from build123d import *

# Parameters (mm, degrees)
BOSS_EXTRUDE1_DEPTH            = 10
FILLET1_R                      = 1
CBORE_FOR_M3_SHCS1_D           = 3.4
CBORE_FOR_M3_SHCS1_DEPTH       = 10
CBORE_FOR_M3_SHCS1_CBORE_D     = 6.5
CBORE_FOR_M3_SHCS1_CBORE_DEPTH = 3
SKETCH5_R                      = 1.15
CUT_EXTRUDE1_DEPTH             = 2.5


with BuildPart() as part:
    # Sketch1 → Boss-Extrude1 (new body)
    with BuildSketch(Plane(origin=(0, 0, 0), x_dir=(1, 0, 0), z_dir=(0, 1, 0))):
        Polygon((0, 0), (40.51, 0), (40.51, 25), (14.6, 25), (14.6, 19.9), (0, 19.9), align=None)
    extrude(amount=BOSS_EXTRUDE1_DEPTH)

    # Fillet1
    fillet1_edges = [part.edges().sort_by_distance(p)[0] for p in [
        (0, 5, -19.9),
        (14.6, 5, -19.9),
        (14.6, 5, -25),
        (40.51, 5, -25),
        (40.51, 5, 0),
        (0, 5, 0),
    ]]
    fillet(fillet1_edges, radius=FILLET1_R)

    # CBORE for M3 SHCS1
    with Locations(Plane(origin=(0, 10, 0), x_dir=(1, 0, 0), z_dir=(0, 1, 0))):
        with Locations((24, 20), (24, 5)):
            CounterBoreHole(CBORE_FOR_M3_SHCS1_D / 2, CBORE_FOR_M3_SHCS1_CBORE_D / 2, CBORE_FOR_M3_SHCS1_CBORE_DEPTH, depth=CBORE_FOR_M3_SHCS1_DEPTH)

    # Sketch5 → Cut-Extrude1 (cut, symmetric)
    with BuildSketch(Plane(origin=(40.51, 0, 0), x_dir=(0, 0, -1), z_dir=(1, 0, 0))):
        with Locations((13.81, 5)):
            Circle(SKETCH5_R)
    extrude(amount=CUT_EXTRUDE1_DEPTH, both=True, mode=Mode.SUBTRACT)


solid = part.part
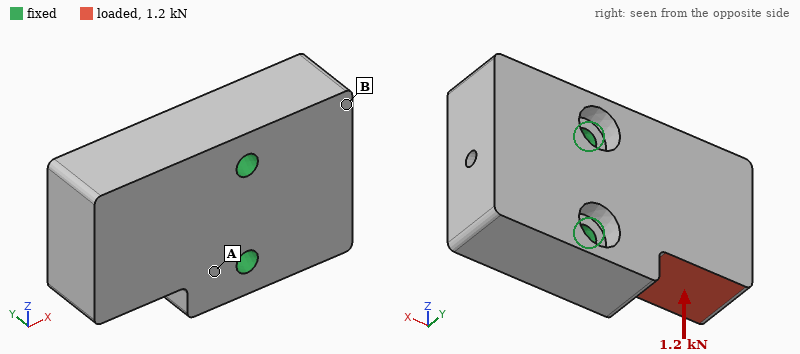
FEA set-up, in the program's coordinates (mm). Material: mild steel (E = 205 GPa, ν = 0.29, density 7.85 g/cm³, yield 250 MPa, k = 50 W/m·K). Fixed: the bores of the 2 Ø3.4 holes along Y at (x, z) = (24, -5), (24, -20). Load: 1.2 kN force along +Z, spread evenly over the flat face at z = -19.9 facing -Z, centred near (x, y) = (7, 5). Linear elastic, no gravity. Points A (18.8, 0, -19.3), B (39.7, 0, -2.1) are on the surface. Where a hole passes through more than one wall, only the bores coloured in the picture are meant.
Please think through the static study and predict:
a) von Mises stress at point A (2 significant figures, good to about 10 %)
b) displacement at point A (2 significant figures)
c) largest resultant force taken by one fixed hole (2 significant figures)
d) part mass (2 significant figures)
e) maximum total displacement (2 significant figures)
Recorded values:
20 MPa
0.62 µm
1.3 kN
71 g
3.7 µm
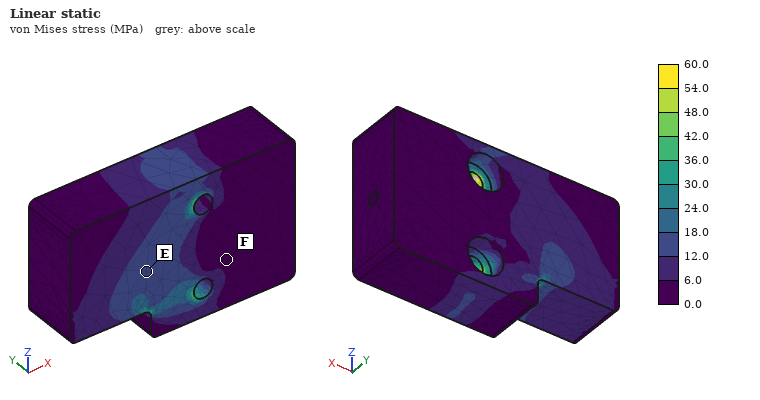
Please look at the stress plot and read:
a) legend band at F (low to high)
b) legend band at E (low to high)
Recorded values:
0.0 to 6.0 MPa
12.0 to 18.0 MPa
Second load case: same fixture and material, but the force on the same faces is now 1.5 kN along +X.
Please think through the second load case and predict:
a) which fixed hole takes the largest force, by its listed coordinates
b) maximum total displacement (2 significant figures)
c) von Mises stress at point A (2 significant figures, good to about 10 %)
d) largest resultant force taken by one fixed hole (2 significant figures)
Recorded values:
(24, -20)
4.1 µm
24 MPa
1.5 kN
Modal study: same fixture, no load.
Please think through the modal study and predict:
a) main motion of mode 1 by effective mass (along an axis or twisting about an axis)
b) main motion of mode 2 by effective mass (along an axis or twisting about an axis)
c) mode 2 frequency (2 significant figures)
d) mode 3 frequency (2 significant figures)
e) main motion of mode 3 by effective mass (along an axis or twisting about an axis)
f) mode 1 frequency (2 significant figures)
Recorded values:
along Y
along Y
20 kHz
21 kHz
along Z
10 kHz
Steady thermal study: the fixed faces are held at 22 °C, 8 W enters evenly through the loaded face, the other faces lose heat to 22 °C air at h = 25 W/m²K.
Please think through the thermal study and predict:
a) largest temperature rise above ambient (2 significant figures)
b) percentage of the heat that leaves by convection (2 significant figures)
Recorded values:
19 K
4.5 %
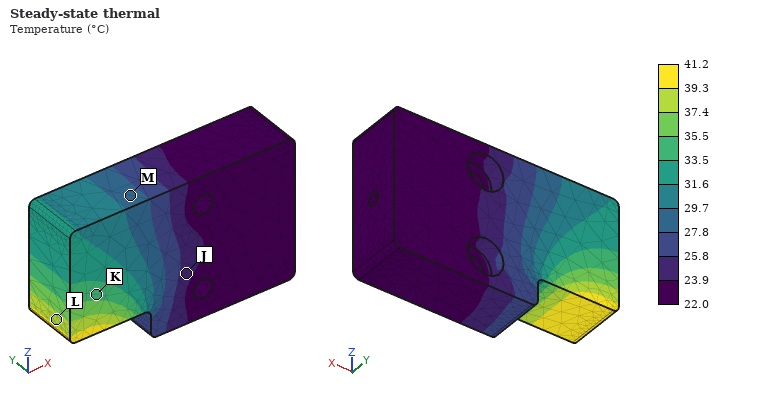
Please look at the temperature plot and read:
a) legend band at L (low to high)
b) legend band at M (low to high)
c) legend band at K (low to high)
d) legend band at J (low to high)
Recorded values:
37.4 to 39.3 °C
27.8 to 29.7 °C
33.5 to 35.5 °C
23.9 to 25.8 °C
